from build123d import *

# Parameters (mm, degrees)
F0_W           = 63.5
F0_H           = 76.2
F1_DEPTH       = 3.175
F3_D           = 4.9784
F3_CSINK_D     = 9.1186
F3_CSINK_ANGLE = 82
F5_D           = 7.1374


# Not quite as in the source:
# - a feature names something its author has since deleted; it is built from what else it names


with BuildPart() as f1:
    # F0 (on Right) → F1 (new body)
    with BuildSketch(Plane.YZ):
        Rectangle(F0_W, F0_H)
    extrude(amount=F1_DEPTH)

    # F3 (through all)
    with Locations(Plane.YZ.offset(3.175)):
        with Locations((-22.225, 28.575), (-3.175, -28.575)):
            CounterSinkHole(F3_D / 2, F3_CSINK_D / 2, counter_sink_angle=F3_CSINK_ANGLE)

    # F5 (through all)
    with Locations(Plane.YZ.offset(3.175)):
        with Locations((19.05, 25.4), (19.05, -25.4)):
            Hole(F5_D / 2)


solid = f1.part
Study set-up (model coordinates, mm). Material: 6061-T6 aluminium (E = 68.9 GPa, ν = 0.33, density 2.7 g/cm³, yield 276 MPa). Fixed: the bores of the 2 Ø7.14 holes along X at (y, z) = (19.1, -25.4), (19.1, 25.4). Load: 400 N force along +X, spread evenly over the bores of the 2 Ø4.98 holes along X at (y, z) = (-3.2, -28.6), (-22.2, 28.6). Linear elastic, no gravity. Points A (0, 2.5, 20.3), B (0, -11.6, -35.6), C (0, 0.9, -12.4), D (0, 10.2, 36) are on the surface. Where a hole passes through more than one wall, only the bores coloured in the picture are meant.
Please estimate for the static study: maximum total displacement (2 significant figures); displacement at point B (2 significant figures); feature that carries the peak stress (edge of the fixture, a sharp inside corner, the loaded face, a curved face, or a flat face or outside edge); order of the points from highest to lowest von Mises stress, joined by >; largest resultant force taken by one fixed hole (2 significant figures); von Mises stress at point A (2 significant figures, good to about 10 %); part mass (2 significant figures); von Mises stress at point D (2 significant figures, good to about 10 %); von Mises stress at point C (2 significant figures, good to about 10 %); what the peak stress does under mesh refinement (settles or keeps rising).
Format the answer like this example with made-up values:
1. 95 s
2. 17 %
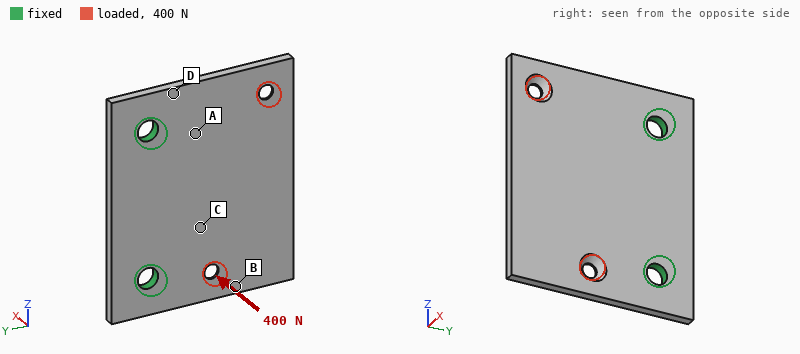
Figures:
1. 0.75 mm
2. 0.22 mm
3. edge of the fixture
4. D > A > C > B
5. 200 N
6. 58 MPa
7. 40 g
8. 91 MPa
9. 31 MPa
10. keeps rising
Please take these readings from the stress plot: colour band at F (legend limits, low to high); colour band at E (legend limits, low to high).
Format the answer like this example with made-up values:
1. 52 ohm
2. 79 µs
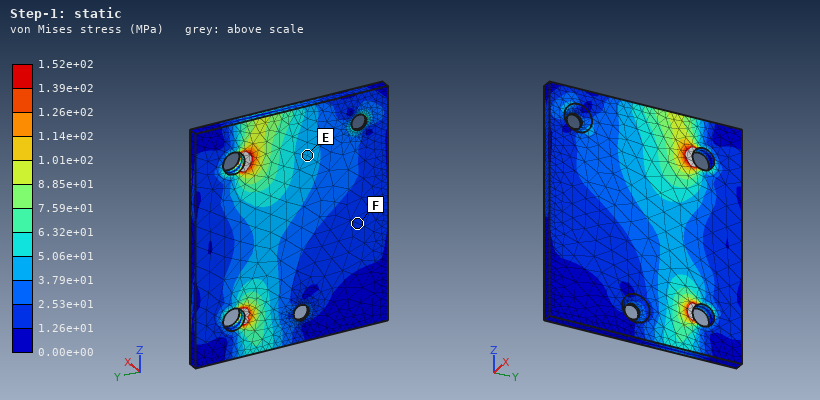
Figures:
1. 1.26e+01 to 2.53e+01 MPa
2. 3.79e+01 to 5.06e+01 MPa
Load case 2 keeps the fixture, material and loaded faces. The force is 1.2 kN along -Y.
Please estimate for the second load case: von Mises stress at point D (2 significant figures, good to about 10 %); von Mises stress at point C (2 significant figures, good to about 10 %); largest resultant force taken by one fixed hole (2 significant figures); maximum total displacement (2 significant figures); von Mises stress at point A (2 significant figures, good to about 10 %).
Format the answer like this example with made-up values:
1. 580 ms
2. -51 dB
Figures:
1. 16 MPa
2. 10.0 MPa
3. 600 N
4. 0.12 mm
5. 15 MPa
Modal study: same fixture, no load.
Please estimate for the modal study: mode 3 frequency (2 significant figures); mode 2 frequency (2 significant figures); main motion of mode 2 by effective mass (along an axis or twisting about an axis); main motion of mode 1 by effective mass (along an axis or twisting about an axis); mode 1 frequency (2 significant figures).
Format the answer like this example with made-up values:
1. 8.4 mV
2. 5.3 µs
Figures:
1. 4000 Hz
2. 1900 Hz
3. twisting about Y
4. along X
5. 1000 Hz
